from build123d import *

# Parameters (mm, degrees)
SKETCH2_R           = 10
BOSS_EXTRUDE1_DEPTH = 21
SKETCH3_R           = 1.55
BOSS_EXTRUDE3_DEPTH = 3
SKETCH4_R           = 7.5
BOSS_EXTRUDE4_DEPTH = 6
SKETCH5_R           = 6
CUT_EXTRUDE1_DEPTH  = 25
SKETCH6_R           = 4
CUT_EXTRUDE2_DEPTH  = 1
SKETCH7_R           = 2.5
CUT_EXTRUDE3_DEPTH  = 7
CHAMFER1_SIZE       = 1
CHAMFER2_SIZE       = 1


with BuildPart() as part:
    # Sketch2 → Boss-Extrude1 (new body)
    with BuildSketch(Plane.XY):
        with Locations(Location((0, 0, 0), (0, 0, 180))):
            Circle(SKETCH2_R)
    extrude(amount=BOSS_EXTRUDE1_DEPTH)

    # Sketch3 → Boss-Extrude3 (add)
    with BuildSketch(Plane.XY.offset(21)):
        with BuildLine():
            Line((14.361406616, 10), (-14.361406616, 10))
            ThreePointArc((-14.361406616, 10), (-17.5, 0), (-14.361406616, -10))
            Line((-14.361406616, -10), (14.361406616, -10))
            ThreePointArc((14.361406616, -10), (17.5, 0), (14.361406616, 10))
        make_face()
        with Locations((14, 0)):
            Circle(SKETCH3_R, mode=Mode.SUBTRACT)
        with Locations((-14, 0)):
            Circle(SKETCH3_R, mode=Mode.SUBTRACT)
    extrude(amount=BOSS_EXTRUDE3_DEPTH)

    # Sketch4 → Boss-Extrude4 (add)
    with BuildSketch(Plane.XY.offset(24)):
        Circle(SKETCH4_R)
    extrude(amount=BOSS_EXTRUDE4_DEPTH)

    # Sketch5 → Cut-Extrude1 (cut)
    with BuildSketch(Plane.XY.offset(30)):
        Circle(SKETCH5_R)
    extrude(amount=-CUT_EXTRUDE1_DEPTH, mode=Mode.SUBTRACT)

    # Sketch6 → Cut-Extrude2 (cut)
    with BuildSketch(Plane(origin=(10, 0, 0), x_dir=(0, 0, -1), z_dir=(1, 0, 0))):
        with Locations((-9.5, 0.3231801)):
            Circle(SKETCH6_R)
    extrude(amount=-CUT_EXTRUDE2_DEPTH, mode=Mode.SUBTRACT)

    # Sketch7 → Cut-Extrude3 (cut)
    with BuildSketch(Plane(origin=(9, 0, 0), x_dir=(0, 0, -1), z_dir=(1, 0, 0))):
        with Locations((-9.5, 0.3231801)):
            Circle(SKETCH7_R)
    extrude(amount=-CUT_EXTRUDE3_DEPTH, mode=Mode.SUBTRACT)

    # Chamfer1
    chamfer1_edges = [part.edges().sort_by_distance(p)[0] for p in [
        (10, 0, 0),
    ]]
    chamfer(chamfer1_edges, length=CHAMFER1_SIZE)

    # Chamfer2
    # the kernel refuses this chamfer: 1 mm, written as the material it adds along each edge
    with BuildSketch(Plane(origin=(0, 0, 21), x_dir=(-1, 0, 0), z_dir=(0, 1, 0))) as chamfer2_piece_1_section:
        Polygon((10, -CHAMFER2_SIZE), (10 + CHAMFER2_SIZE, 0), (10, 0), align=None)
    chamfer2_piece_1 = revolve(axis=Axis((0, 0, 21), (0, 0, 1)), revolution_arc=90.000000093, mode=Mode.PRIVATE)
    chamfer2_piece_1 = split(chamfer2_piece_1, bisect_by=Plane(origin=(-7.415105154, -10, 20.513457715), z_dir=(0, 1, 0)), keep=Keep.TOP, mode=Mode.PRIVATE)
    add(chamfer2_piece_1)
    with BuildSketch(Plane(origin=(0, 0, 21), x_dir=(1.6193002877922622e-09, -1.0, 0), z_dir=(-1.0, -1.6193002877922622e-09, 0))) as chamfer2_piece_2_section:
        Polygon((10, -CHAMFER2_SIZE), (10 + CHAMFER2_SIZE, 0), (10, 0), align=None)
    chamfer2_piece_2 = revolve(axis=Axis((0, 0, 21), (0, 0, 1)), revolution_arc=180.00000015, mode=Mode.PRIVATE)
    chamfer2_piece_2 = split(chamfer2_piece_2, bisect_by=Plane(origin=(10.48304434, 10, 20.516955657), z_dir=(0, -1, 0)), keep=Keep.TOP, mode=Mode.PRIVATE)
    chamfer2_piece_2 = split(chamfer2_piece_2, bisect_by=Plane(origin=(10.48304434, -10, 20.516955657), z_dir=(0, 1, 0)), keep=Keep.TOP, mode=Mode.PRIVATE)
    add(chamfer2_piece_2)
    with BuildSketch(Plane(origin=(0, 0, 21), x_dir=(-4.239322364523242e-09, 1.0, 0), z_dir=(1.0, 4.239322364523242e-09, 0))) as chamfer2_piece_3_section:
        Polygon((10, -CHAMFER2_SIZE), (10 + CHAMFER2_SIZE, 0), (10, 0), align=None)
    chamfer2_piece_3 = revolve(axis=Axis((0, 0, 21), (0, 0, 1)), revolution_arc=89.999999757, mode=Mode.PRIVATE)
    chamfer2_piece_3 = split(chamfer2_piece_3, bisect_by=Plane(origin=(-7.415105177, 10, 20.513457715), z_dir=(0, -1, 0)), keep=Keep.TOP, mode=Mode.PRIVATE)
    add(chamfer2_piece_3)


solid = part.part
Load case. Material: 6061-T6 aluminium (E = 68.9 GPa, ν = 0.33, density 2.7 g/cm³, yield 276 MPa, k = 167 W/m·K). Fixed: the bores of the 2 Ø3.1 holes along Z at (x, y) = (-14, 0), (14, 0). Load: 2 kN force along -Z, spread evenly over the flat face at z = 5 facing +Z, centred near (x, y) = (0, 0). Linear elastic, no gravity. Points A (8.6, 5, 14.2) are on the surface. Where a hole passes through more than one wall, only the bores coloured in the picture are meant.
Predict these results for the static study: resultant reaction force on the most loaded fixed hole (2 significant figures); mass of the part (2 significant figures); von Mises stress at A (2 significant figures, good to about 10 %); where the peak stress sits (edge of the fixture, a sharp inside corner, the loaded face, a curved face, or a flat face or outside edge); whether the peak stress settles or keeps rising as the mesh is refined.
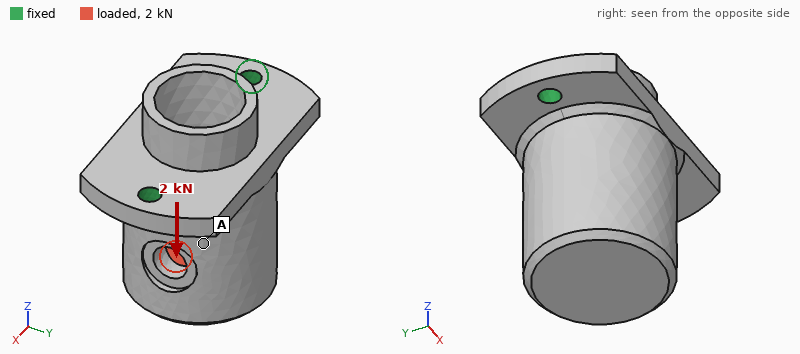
1.1 kN
18 g
25 MPa
edge of the fixture
keeps rising
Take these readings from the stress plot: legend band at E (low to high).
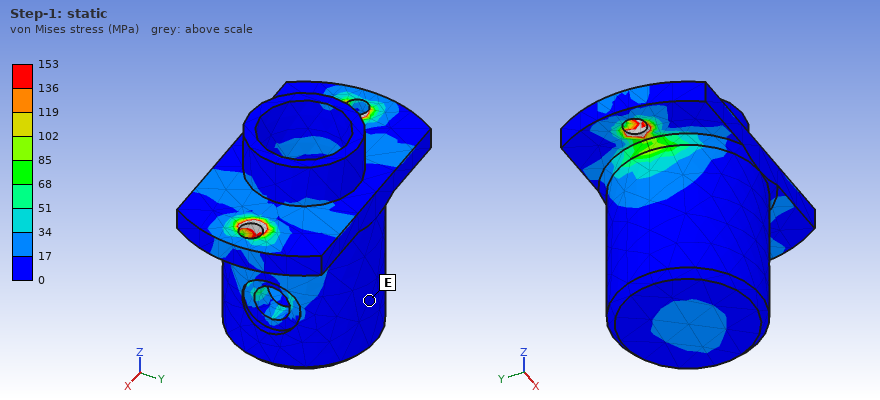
0 to 17 MPa
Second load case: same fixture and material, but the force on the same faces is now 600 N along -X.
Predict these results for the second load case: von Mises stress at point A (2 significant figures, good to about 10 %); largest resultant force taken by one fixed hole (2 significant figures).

10 MPa
540 N
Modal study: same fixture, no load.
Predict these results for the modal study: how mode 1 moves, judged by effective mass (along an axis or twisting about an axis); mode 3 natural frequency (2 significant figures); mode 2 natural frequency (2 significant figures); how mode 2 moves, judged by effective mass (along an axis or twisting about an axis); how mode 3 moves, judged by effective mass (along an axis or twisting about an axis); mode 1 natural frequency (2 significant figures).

along Y
14 kHz
11 kHz
along X
along Z
3500 Hz
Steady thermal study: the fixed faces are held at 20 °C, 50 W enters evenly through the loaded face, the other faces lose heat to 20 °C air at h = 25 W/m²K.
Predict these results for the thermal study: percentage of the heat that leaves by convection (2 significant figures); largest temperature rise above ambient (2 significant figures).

5.5 %
58 K
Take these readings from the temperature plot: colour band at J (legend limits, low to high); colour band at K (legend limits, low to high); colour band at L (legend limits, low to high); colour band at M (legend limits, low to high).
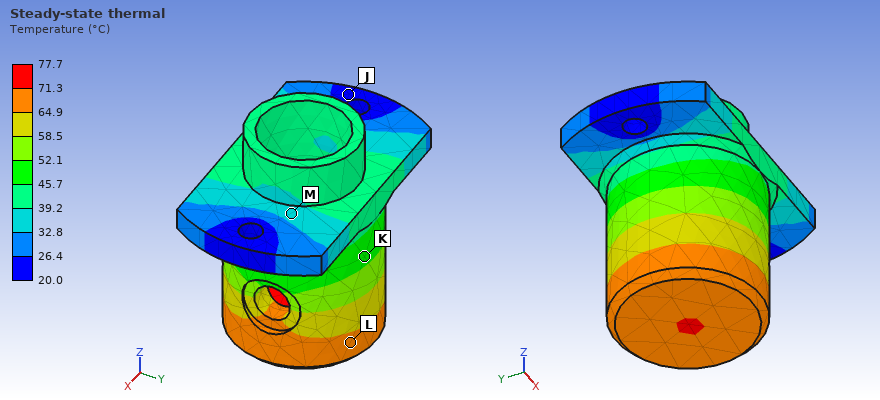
20.0 to 26.4 °C
45.7 to 52.1 °C
64.9 to 71.3 °C
32.8 to 39.2 °C
